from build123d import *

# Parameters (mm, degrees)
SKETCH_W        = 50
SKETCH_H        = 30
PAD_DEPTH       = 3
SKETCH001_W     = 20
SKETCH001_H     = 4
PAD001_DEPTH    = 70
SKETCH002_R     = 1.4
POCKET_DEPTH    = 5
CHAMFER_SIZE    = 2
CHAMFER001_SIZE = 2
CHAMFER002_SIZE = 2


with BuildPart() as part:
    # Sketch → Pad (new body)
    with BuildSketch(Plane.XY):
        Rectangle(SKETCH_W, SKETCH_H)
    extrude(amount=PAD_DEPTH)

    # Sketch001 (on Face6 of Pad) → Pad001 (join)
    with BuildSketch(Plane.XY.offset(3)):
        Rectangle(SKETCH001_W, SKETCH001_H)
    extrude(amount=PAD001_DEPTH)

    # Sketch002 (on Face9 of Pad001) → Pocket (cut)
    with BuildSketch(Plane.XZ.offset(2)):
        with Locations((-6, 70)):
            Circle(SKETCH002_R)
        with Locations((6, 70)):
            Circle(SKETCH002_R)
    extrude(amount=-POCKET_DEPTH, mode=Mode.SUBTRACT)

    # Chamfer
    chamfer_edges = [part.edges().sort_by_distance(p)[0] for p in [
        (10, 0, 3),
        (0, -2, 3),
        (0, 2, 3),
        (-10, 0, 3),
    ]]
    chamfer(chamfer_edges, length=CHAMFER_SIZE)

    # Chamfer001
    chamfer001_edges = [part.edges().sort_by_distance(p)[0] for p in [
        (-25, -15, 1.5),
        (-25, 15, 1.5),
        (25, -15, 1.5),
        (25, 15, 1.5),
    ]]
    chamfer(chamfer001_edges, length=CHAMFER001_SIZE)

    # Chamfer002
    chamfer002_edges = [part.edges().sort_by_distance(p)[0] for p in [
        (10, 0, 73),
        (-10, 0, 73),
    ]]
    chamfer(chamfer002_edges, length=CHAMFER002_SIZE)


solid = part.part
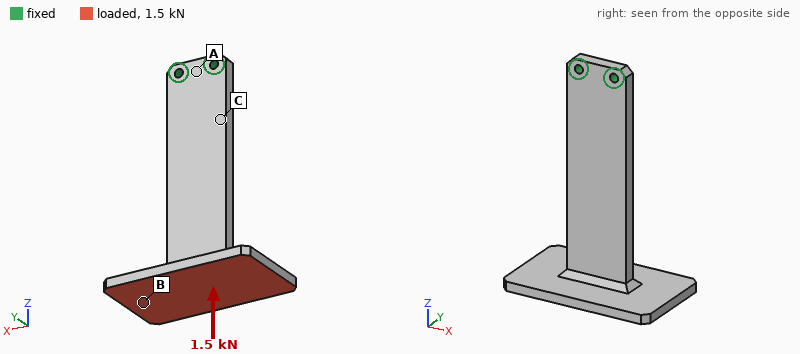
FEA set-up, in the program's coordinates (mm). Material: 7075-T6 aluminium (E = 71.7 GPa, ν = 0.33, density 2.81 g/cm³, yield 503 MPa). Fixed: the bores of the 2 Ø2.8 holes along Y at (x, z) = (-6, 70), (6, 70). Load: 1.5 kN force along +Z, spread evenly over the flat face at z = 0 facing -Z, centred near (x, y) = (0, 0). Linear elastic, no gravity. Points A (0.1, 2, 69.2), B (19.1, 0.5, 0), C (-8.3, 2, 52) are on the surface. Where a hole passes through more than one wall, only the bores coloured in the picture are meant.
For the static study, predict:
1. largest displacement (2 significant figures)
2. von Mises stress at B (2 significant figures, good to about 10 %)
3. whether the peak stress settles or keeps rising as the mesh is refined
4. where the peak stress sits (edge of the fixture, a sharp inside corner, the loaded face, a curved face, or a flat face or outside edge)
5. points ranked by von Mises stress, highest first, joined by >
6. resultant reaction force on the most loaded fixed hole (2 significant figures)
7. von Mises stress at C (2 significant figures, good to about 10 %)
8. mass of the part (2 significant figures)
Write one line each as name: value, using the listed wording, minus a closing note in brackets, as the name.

largest displacement: 99 µm
von Mises stress at B: 30 MPa
whether the peak stress settles or keeps rising as the mesh is refined: keeps rising
where the peak stress sits: a sharp inside corner
points ranked by von Mises stress, highest first, joined by >: B > C > A
resultant reaction force on the most loaded fixed hole: 760 N
von Mises stress at C: 19 MPa
mass of the part: 28 g
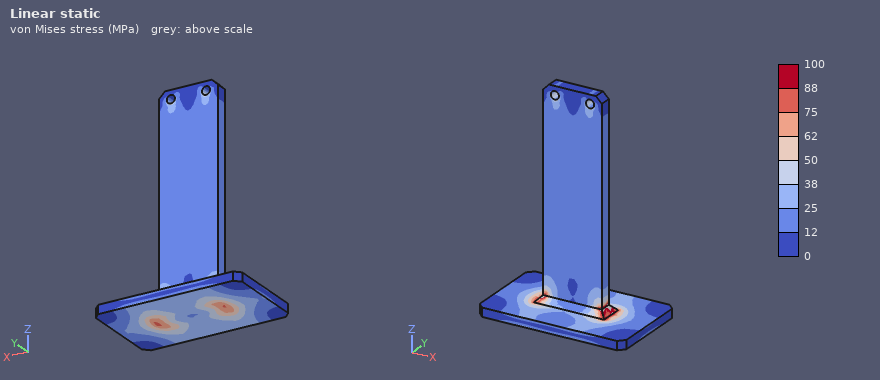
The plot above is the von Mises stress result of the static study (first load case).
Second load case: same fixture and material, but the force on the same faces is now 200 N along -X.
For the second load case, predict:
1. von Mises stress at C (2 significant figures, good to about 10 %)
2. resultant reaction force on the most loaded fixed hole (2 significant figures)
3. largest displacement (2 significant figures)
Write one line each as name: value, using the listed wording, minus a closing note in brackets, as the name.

von Mises stress at C: 32 MPa
resultant reaction force on the most loaded fixed hole: 1.0 kN
largest displacement: 0.15 mm
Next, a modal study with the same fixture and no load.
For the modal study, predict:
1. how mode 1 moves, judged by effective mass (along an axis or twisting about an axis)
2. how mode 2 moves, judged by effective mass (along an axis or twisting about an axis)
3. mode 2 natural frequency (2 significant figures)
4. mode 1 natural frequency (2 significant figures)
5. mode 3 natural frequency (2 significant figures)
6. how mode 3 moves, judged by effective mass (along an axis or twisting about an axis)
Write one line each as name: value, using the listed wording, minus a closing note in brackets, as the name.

how mode 1 moves, judged by effective mass: along Y
how mode 2 moves, judged by effective mass: twisting about Z
mode 2 natural frequency: 1100 Hz
mode 1 natural frequency: 330 Hz
mode 3 natural frequency: 1500 Hz
how mode 3 moves, judged by effective mass: along X
